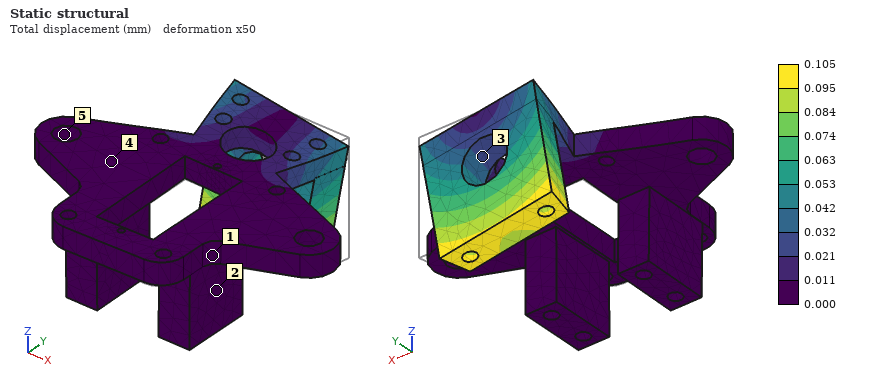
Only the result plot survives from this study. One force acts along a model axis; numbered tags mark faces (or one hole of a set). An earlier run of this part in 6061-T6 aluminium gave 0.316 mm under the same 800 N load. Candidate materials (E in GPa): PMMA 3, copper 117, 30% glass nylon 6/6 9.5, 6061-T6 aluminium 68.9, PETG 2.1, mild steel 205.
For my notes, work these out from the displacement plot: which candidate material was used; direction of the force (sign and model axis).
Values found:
mild steel
-X
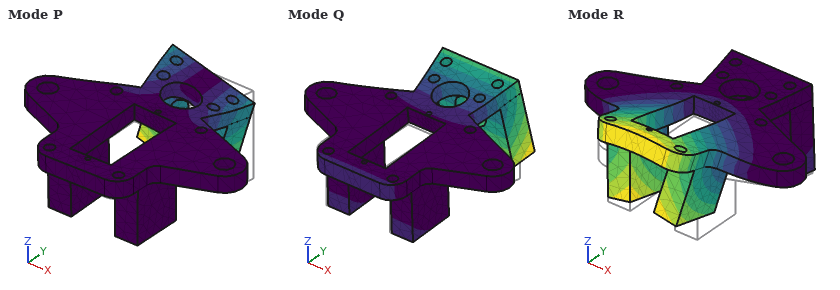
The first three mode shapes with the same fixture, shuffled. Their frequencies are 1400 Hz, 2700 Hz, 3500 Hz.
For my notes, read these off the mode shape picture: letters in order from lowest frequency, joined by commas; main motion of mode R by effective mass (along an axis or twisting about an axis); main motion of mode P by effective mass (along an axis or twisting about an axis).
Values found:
Q, P, R
along Z
along X
